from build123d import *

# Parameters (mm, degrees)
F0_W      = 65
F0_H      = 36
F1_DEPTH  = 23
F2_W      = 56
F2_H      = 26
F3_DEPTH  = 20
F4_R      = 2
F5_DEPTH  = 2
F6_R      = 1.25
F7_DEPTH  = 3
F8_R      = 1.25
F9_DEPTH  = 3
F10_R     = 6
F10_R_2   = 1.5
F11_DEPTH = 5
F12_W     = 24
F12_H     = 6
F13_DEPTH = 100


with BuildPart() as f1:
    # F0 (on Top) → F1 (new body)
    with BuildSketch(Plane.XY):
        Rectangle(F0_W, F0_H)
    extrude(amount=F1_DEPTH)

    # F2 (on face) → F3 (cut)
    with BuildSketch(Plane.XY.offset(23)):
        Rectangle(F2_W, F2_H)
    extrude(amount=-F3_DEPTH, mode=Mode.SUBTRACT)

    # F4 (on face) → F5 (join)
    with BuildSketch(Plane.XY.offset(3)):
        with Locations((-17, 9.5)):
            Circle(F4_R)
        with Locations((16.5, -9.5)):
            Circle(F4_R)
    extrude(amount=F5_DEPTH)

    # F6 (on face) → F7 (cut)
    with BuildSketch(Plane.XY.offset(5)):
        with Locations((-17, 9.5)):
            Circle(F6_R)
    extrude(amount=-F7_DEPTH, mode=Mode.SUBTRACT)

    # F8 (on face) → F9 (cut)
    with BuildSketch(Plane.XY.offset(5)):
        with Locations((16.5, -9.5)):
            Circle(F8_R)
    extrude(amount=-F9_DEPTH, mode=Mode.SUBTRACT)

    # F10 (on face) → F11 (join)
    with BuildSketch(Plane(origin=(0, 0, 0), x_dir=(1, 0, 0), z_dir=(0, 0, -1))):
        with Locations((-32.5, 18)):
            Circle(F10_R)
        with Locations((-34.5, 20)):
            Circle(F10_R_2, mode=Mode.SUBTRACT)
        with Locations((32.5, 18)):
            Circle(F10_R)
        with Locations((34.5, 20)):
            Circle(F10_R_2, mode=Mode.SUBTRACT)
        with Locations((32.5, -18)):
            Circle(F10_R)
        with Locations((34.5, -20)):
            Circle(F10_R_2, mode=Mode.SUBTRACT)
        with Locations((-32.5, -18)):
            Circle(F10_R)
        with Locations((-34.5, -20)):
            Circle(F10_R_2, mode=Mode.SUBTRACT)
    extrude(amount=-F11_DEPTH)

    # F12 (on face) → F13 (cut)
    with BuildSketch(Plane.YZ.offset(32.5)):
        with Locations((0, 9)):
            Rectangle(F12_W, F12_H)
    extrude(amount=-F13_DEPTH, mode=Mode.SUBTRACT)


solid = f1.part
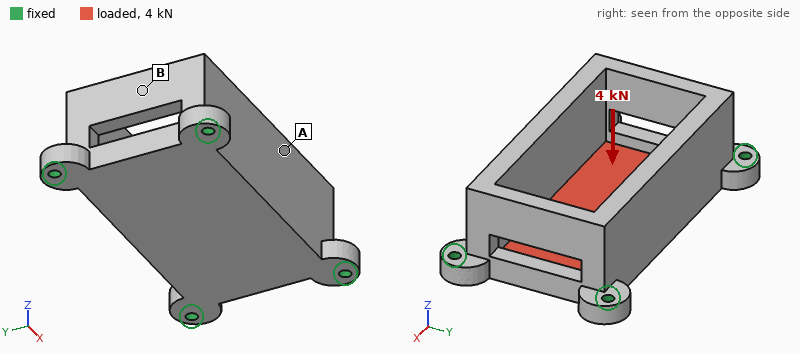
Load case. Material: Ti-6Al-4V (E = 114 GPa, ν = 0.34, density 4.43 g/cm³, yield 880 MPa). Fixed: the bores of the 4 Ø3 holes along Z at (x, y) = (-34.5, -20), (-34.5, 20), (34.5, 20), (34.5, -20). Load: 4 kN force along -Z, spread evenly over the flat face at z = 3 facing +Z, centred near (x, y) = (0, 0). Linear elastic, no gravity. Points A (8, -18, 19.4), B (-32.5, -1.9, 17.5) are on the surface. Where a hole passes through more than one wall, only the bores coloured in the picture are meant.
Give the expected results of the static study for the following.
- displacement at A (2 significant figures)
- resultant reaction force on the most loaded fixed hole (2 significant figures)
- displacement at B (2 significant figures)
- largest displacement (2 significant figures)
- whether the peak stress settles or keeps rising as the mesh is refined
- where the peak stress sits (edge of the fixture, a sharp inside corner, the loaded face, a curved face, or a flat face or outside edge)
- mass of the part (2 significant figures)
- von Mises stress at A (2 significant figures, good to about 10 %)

25 µm
1.1 kN
7.5 µm
49 µm
keeps rising
edge of the fixture
110 g
36 MPa
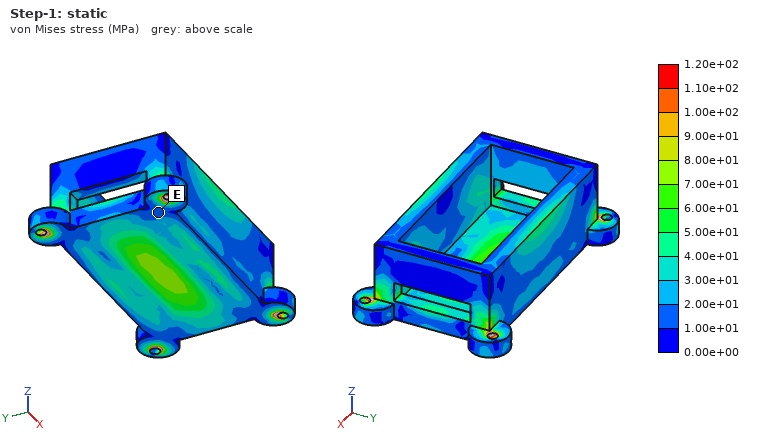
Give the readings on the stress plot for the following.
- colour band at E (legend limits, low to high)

1.00e+01 to 2.00e+01 MPa
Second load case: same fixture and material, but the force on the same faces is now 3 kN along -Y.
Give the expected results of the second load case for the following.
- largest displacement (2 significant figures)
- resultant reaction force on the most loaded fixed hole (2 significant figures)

8.3 µm
960 N
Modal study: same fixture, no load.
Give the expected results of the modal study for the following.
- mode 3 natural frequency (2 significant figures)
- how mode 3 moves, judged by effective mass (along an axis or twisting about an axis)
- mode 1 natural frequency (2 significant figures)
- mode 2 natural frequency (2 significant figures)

9200 Hz
along Z
7300 Hz
7400 Hz
